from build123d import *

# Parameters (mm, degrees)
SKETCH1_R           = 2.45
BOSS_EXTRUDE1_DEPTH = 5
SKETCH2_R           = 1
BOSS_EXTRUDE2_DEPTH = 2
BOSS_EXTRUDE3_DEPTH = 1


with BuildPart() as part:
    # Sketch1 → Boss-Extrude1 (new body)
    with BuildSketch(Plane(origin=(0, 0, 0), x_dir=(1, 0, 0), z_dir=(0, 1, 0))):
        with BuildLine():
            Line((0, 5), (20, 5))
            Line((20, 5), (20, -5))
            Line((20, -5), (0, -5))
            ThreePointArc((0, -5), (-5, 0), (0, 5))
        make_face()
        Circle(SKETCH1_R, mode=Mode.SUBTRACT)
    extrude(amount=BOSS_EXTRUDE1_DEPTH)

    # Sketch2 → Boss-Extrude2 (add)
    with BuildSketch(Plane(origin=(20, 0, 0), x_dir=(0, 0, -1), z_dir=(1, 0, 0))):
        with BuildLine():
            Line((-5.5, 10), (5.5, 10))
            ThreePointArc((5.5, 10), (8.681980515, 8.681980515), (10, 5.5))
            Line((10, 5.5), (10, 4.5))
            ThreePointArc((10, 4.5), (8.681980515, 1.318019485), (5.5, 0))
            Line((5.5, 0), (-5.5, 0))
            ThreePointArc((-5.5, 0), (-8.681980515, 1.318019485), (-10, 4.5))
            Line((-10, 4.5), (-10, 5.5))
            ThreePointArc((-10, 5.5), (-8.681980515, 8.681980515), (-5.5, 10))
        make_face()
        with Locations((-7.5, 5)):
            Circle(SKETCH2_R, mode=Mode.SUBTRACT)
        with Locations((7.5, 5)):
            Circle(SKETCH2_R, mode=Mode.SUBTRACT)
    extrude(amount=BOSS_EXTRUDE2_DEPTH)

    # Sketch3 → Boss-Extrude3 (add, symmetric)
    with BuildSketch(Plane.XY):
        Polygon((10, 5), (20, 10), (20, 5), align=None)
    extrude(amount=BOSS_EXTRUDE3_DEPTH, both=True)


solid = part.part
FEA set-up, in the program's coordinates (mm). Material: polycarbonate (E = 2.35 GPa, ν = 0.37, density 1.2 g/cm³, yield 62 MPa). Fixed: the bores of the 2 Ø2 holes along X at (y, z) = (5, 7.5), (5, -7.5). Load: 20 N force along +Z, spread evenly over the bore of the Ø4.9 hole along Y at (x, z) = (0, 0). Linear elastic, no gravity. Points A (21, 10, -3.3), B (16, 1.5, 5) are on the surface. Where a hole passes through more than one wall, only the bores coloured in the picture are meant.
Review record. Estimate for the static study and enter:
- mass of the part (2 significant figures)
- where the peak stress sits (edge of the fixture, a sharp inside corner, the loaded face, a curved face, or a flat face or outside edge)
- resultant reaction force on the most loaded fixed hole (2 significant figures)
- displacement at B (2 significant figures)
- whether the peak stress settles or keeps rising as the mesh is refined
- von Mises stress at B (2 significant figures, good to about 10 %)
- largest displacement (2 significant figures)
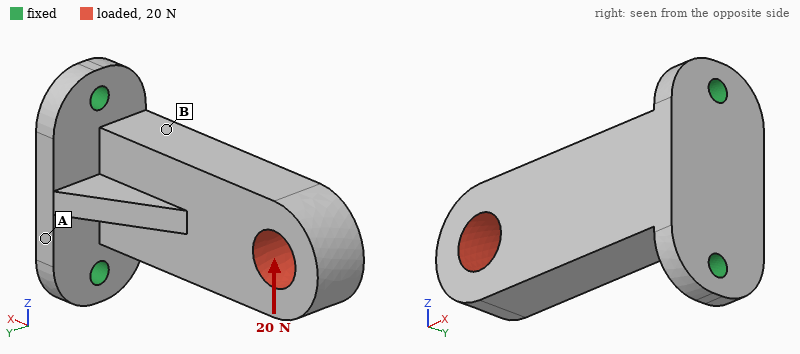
1.8 g
edge of the fixture
36 N
0.041 mm
keeps rising
3.5 MPa
0.21 mm
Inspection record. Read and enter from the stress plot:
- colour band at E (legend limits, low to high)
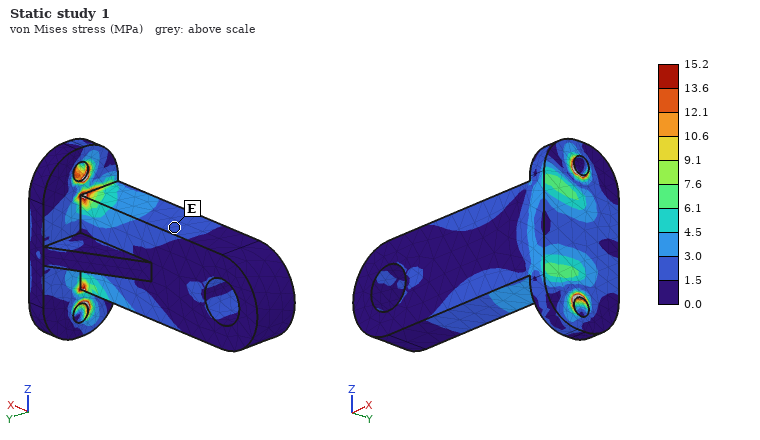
1.5 to 3.0 MPa
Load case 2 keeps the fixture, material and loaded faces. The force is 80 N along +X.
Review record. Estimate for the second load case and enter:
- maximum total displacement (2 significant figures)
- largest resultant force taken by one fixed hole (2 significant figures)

0.37 mm
42 N
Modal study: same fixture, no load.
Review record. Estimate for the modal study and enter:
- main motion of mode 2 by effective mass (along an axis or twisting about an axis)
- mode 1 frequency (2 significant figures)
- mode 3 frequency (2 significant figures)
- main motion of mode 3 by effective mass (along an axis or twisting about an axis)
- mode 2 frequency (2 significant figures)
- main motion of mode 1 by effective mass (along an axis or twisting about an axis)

along Z
960 Hz
5700 Hz
along X
2300 Hz
along Y
